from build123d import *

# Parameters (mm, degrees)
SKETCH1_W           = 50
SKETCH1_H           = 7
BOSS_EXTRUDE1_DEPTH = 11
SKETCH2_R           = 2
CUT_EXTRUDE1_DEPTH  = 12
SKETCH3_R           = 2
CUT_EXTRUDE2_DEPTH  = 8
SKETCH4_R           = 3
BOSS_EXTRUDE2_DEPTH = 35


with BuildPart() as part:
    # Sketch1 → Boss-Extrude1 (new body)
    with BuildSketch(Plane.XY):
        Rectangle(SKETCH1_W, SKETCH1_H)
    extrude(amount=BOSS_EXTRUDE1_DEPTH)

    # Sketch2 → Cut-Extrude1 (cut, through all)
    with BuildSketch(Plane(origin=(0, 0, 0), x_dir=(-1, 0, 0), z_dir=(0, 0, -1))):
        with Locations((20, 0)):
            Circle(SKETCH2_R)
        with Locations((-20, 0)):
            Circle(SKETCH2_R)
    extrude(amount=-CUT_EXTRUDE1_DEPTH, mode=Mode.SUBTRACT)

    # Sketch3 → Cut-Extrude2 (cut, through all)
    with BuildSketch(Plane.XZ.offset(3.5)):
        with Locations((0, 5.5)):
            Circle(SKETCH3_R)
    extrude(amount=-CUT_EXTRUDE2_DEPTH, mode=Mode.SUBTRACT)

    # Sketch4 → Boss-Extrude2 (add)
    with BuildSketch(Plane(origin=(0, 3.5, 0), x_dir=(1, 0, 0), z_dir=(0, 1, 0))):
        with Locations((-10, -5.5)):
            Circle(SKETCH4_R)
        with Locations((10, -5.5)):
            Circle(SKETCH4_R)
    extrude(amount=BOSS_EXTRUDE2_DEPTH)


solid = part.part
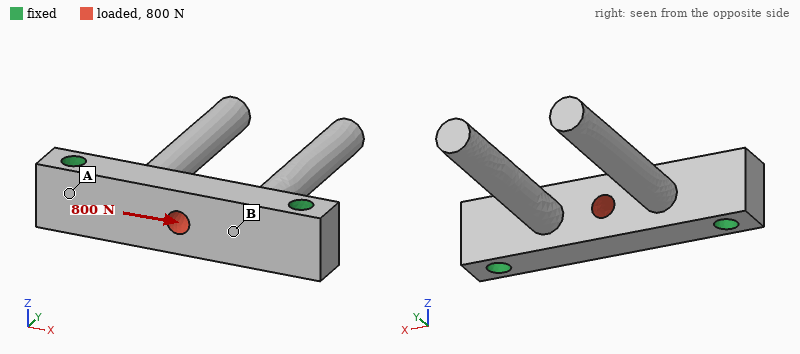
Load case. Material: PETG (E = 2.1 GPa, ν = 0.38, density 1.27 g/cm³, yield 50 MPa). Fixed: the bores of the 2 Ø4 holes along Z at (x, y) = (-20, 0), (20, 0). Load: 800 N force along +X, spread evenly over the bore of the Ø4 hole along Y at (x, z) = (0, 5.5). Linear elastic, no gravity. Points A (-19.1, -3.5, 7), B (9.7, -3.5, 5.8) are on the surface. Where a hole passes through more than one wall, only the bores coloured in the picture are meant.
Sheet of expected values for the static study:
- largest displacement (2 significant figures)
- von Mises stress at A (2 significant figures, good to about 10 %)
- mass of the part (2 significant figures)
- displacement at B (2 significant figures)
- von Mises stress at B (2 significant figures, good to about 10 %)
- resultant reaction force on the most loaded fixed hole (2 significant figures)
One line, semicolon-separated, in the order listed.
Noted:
51 µm; 2.4 MPa; 6.9 g; 22 µm; 6.0 MPa; 400 N
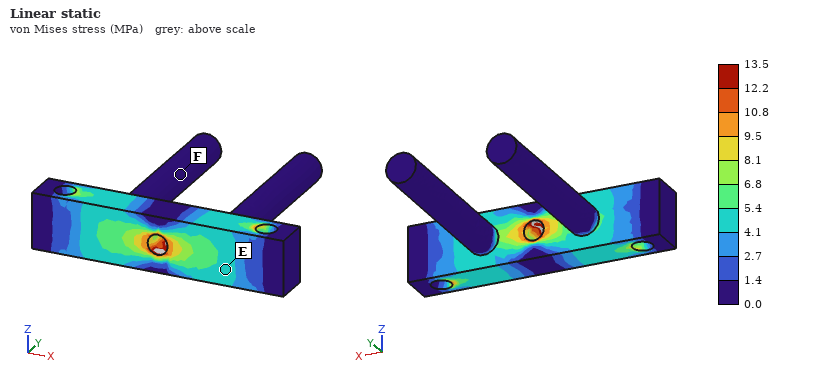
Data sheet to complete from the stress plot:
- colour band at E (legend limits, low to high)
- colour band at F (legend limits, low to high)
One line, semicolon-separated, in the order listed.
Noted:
4.1 to 5.4 MPa; 0.0 to 1.4 MPa
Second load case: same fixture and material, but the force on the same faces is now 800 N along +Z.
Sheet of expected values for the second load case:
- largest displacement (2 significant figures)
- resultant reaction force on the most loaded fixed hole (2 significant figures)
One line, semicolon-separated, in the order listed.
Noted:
0.28 mm; 400 N
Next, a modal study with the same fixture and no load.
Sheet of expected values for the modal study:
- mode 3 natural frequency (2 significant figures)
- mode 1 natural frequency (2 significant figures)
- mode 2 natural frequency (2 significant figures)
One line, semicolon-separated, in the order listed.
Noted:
780 Hz; 740 Hz; 770 Hz
